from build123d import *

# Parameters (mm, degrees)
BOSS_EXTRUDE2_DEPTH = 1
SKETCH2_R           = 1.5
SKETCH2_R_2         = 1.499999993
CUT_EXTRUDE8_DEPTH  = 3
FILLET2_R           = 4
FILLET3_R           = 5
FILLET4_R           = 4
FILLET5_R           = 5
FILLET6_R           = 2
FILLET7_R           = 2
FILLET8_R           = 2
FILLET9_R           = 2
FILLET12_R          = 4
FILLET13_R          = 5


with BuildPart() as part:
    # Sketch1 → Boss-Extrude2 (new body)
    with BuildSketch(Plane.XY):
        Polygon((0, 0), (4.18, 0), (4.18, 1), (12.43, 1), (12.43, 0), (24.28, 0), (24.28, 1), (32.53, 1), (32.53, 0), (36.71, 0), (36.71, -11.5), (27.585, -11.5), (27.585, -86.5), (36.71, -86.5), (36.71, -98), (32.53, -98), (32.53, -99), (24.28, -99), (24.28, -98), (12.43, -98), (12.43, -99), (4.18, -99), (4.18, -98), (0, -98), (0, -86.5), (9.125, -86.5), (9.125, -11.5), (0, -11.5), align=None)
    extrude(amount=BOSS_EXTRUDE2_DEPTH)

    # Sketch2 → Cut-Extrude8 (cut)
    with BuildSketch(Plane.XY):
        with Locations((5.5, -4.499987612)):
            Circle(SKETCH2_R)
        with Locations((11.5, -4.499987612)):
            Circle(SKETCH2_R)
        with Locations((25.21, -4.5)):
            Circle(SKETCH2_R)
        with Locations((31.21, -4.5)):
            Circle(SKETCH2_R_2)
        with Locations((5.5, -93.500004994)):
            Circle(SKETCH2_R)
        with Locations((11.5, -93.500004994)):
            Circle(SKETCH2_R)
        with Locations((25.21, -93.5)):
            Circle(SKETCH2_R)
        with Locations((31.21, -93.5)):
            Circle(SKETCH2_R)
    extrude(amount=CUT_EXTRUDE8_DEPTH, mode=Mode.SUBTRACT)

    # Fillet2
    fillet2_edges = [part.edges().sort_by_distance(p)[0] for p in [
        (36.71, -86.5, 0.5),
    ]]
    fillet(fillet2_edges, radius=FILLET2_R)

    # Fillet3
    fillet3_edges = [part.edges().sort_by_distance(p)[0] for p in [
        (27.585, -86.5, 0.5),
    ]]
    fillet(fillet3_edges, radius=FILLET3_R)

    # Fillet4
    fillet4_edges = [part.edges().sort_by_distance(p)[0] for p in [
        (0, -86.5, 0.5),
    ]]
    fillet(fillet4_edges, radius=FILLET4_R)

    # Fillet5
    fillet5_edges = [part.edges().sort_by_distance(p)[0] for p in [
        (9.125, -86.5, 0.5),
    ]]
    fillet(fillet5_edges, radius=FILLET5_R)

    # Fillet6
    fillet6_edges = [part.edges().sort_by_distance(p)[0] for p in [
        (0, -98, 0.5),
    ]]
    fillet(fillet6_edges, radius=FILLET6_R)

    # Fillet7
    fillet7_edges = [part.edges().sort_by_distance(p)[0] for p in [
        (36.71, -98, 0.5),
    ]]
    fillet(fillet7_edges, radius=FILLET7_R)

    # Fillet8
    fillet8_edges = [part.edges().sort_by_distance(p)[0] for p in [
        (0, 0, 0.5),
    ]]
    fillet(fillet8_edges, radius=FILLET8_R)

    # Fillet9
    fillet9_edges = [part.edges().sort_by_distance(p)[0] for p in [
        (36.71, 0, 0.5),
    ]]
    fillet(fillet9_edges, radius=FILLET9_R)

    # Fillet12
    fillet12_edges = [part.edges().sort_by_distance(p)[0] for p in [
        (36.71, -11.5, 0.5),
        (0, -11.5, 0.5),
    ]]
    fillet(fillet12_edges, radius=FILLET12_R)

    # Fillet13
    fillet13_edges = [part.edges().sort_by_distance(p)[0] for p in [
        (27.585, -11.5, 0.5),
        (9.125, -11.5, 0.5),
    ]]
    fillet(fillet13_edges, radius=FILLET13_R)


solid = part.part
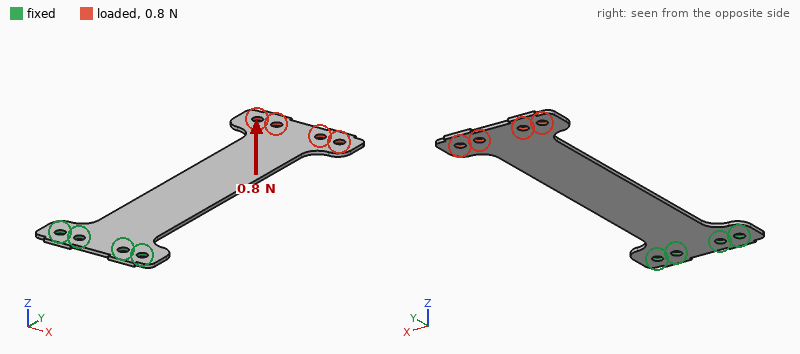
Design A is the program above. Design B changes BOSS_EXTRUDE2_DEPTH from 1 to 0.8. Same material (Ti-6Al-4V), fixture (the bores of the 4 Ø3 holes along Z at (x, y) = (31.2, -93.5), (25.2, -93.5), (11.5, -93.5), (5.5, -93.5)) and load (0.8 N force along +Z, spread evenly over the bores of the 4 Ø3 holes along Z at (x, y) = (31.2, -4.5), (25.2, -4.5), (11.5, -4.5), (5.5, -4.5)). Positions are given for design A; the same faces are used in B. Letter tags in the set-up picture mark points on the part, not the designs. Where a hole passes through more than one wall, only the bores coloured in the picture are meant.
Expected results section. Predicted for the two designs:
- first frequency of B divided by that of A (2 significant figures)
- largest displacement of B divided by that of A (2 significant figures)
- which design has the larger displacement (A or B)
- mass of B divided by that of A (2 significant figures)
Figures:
0.80
2.0
B
0.80
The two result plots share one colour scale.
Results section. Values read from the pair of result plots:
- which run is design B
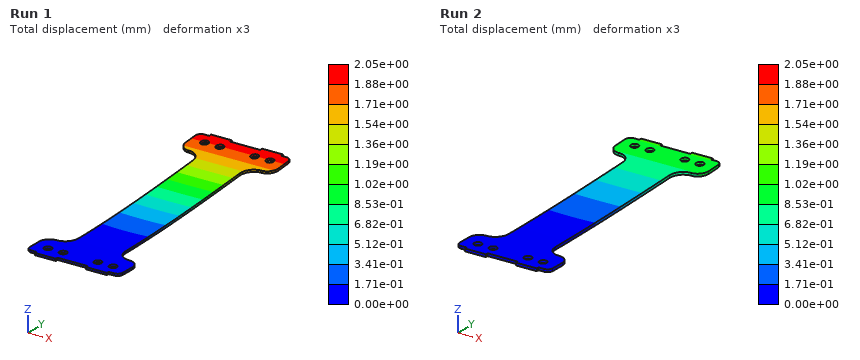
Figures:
Run 1
